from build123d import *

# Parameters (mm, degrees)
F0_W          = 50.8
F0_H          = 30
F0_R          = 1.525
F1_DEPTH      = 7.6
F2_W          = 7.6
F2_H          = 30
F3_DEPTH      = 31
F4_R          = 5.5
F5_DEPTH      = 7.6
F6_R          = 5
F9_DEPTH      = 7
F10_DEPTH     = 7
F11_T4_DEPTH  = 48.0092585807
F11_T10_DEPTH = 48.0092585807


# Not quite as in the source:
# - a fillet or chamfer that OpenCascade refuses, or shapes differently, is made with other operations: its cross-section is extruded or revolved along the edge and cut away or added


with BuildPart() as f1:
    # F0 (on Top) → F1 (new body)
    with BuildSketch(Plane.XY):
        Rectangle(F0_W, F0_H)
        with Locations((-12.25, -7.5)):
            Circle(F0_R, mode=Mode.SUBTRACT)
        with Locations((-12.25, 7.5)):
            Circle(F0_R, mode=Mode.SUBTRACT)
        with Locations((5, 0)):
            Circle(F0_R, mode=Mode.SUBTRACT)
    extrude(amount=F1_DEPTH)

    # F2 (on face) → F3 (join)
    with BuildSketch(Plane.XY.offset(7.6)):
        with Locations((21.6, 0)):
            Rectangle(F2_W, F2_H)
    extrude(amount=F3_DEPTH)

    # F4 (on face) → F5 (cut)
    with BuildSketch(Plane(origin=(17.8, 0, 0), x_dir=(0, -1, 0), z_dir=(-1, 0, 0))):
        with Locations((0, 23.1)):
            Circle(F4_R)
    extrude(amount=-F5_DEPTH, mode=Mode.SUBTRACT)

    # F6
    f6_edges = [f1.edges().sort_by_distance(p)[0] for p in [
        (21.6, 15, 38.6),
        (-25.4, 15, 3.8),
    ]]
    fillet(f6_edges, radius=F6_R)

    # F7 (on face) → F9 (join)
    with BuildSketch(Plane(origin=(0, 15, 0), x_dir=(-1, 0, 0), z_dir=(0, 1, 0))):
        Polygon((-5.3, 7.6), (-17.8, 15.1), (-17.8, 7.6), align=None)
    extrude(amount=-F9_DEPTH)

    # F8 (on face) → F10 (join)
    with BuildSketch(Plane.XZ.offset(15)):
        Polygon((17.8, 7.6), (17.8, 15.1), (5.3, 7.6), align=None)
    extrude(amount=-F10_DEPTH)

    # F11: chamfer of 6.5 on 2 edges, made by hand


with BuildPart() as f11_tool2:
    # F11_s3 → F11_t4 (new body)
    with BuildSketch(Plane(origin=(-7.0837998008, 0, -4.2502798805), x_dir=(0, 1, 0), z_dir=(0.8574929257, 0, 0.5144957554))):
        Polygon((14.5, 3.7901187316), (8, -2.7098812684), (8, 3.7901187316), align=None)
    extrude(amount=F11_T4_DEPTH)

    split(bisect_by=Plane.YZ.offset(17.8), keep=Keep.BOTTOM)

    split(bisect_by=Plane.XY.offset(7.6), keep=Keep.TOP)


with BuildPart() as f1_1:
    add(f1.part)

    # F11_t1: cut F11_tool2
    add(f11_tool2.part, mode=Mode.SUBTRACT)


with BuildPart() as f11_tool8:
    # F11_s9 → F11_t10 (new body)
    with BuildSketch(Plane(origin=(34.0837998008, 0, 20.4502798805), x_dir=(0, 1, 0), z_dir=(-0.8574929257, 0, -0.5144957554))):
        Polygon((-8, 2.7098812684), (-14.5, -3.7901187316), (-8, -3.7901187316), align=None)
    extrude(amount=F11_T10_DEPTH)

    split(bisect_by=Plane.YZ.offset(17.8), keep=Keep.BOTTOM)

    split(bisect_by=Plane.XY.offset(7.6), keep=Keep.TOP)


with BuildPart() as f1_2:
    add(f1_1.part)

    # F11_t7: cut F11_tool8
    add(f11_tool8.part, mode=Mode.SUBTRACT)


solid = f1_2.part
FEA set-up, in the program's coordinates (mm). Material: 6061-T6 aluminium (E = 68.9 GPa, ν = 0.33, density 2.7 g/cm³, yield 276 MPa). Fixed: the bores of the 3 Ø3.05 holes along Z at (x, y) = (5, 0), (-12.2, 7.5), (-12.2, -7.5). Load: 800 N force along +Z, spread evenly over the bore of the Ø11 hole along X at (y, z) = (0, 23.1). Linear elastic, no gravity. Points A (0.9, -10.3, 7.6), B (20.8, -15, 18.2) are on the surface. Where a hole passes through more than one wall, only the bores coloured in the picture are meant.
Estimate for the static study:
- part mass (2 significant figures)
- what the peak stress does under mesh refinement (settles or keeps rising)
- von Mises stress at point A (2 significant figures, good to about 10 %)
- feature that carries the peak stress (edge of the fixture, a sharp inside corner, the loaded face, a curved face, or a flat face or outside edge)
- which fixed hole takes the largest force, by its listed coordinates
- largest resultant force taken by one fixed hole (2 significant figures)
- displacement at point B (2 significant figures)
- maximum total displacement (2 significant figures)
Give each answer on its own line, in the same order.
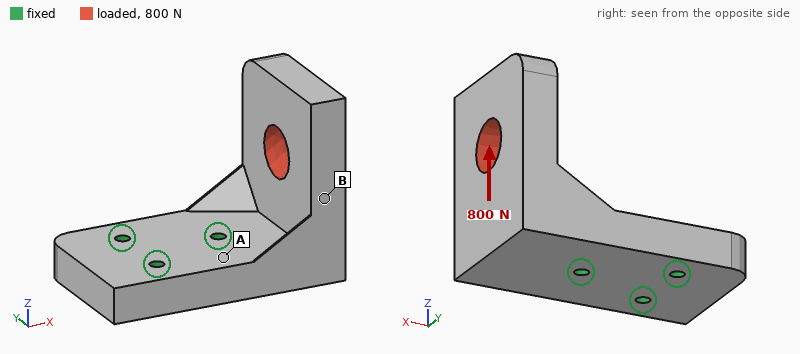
48 g
keeps rising
19 MPa
edge of the fixture
(5, 0)
1.2 kN
34 µm
68 µm
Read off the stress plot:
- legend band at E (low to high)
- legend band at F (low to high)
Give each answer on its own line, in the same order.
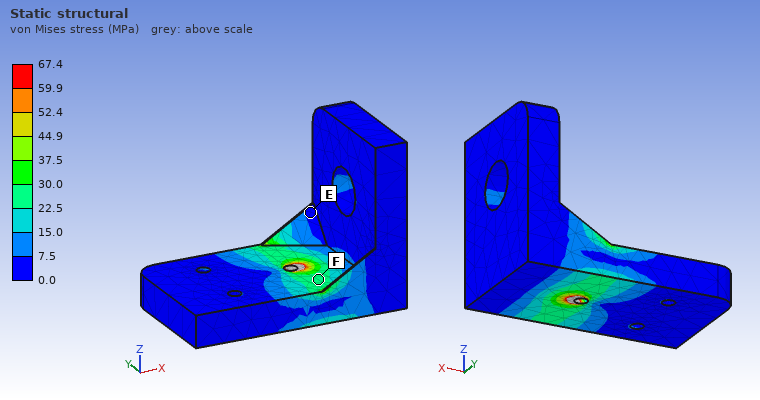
0.0 to 7.5 MPa
22.5 to 30.0 MPa
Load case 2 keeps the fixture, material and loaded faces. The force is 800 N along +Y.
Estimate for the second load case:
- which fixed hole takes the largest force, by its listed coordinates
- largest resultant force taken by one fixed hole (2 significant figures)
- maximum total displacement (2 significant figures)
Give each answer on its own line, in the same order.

(5, 0)
1.1 kN
97 µm
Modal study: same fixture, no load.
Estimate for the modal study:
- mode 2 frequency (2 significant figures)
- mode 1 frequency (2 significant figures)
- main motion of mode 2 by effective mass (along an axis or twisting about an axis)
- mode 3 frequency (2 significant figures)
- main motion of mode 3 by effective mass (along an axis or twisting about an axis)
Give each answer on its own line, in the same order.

4000 Hz
3200 Hz
along Y
8700 Hz
along Z
